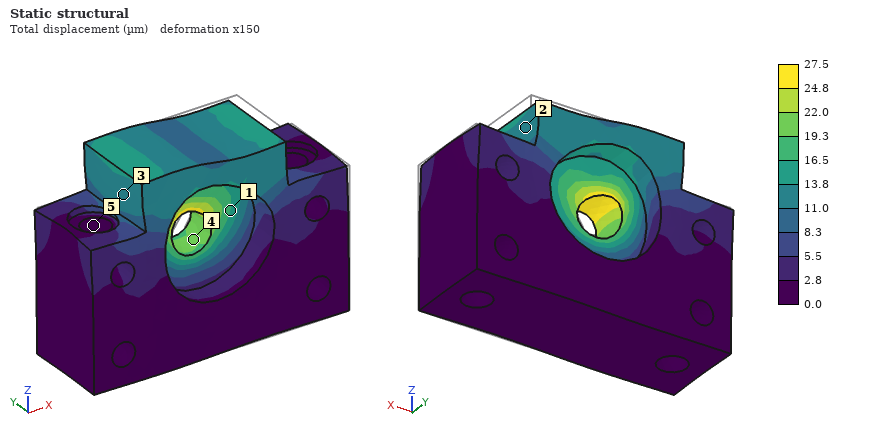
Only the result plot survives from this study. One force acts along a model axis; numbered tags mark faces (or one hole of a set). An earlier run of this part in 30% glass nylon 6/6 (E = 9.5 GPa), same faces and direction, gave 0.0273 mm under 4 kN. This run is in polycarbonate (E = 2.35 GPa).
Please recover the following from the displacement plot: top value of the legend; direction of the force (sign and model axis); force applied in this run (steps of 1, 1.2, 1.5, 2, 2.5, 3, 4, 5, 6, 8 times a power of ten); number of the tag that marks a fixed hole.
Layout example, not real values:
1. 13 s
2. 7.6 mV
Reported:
1. 27.5 µm
2. -X
3. 1 kN
4. 5
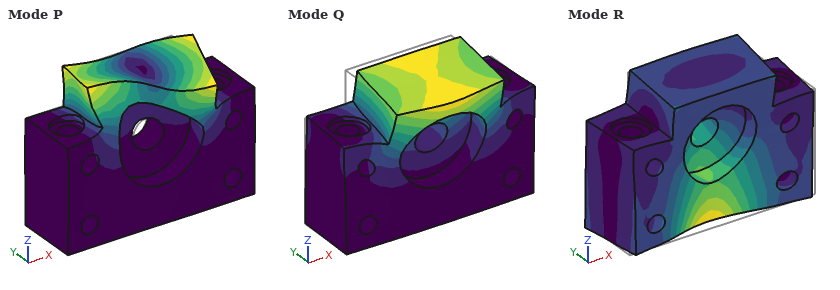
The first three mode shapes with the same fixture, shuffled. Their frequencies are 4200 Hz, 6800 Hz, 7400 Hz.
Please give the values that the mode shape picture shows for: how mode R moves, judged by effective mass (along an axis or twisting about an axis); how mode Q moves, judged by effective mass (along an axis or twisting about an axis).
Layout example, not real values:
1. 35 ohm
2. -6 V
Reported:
1. along Y
2. along Y
